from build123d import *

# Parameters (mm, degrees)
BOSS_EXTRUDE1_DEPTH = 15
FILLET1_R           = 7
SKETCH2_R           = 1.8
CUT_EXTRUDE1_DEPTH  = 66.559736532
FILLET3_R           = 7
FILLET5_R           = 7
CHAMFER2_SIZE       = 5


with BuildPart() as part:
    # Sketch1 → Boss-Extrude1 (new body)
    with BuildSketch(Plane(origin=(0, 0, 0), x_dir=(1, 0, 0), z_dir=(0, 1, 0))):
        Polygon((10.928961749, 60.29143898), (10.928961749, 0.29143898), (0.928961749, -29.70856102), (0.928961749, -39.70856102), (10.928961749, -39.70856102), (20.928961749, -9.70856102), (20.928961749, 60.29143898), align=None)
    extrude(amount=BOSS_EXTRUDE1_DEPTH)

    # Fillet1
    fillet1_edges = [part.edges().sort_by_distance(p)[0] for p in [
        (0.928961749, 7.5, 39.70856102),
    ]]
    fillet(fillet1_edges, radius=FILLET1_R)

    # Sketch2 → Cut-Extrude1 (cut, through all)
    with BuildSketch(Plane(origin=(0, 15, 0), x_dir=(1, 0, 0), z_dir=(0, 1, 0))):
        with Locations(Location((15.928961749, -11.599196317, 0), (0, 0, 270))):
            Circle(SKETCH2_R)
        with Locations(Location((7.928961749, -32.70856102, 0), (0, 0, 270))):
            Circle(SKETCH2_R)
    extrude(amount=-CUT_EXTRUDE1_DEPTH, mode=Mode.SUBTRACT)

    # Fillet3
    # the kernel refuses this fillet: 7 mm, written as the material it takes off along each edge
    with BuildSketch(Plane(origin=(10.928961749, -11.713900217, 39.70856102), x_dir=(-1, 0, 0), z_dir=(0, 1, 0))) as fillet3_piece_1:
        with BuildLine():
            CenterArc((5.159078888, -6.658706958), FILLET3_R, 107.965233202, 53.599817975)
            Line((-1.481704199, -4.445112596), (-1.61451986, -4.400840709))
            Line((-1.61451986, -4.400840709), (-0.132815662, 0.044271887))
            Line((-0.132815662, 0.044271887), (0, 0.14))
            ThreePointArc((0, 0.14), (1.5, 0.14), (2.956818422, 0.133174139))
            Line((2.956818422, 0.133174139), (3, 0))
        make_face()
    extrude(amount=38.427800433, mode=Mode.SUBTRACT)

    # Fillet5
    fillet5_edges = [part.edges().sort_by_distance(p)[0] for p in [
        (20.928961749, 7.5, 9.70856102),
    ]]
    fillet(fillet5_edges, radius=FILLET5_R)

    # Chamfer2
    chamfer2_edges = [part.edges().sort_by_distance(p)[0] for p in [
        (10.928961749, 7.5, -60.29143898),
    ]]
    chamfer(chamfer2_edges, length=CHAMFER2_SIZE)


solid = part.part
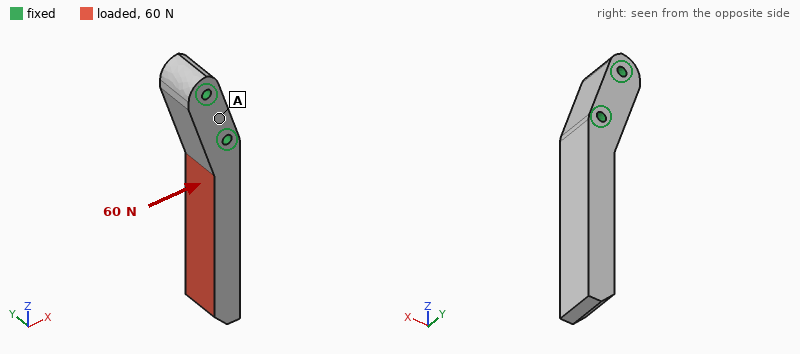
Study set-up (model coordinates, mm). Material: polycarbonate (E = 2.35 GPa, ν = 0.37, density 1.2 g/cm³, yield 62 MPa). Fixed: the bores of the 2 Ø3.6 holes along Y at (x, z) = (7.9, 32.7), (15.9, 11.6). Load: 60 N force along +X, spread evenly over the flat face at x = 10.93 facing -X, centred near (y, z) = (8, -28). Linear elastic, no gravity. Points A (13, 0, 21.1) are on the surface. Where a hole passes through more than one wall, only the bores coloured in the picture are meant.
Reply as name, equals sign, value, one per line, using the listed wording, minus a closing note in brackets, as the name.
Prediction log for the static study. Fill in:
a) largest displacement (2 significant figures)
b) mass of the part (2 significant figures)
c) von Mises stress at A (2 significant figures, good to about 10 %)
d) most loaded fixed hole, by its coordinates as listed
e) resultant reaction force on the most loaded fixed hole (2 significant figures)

largest displacement = 0.94 mm
mass of the part = 19 g
von Mises stress at A = 0.76 MPa
most loaded fixed hole, by its coordinates as listed = (15.9, 11.6)
resultant reaction force on the most loaded fixed hole = 130 N
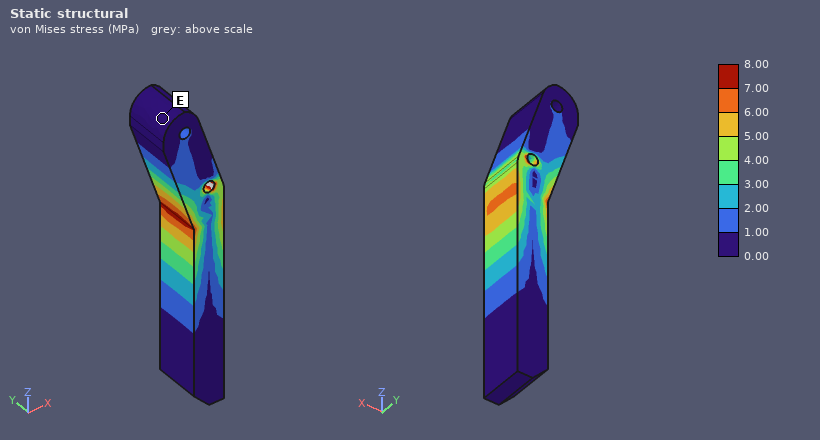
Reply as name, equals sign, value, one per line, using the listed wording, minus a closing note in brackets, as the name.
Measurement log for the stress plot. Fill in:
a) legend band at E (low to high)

legend band at E = 0.00 to 1.00 MPa
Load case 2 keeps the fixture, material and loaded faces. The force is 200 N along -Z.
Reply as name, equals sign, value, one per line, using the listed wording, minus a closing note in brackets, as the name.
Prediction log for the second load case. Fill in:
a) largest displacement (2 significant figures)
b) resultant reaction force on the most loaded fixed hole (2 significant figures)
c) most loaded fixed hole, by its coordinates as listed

largest displacement = 0.58 mm
resultant reaction force on the most loaded fixed hole = 150 N
most loaded fixed hole, by its coordinates as listed = (15.9, 11.6)
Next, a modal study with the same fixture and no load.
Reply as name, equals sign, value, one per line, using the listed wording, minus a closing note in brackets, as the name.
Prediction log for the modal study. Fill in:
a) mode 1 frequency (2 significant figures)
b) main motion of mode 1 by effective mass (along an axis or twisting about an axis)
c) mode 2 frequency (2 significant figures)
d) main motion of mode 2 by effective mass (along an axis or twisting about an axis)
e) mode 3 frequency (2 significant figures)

mode 1 frequency = 470 Hz
main motion of mode 1 by effective mass = along X
mode 2 frequency = 670 Hz
main motion of mode 2 by effective mass = along Y
mode 3 frequency = 2600 Hz
